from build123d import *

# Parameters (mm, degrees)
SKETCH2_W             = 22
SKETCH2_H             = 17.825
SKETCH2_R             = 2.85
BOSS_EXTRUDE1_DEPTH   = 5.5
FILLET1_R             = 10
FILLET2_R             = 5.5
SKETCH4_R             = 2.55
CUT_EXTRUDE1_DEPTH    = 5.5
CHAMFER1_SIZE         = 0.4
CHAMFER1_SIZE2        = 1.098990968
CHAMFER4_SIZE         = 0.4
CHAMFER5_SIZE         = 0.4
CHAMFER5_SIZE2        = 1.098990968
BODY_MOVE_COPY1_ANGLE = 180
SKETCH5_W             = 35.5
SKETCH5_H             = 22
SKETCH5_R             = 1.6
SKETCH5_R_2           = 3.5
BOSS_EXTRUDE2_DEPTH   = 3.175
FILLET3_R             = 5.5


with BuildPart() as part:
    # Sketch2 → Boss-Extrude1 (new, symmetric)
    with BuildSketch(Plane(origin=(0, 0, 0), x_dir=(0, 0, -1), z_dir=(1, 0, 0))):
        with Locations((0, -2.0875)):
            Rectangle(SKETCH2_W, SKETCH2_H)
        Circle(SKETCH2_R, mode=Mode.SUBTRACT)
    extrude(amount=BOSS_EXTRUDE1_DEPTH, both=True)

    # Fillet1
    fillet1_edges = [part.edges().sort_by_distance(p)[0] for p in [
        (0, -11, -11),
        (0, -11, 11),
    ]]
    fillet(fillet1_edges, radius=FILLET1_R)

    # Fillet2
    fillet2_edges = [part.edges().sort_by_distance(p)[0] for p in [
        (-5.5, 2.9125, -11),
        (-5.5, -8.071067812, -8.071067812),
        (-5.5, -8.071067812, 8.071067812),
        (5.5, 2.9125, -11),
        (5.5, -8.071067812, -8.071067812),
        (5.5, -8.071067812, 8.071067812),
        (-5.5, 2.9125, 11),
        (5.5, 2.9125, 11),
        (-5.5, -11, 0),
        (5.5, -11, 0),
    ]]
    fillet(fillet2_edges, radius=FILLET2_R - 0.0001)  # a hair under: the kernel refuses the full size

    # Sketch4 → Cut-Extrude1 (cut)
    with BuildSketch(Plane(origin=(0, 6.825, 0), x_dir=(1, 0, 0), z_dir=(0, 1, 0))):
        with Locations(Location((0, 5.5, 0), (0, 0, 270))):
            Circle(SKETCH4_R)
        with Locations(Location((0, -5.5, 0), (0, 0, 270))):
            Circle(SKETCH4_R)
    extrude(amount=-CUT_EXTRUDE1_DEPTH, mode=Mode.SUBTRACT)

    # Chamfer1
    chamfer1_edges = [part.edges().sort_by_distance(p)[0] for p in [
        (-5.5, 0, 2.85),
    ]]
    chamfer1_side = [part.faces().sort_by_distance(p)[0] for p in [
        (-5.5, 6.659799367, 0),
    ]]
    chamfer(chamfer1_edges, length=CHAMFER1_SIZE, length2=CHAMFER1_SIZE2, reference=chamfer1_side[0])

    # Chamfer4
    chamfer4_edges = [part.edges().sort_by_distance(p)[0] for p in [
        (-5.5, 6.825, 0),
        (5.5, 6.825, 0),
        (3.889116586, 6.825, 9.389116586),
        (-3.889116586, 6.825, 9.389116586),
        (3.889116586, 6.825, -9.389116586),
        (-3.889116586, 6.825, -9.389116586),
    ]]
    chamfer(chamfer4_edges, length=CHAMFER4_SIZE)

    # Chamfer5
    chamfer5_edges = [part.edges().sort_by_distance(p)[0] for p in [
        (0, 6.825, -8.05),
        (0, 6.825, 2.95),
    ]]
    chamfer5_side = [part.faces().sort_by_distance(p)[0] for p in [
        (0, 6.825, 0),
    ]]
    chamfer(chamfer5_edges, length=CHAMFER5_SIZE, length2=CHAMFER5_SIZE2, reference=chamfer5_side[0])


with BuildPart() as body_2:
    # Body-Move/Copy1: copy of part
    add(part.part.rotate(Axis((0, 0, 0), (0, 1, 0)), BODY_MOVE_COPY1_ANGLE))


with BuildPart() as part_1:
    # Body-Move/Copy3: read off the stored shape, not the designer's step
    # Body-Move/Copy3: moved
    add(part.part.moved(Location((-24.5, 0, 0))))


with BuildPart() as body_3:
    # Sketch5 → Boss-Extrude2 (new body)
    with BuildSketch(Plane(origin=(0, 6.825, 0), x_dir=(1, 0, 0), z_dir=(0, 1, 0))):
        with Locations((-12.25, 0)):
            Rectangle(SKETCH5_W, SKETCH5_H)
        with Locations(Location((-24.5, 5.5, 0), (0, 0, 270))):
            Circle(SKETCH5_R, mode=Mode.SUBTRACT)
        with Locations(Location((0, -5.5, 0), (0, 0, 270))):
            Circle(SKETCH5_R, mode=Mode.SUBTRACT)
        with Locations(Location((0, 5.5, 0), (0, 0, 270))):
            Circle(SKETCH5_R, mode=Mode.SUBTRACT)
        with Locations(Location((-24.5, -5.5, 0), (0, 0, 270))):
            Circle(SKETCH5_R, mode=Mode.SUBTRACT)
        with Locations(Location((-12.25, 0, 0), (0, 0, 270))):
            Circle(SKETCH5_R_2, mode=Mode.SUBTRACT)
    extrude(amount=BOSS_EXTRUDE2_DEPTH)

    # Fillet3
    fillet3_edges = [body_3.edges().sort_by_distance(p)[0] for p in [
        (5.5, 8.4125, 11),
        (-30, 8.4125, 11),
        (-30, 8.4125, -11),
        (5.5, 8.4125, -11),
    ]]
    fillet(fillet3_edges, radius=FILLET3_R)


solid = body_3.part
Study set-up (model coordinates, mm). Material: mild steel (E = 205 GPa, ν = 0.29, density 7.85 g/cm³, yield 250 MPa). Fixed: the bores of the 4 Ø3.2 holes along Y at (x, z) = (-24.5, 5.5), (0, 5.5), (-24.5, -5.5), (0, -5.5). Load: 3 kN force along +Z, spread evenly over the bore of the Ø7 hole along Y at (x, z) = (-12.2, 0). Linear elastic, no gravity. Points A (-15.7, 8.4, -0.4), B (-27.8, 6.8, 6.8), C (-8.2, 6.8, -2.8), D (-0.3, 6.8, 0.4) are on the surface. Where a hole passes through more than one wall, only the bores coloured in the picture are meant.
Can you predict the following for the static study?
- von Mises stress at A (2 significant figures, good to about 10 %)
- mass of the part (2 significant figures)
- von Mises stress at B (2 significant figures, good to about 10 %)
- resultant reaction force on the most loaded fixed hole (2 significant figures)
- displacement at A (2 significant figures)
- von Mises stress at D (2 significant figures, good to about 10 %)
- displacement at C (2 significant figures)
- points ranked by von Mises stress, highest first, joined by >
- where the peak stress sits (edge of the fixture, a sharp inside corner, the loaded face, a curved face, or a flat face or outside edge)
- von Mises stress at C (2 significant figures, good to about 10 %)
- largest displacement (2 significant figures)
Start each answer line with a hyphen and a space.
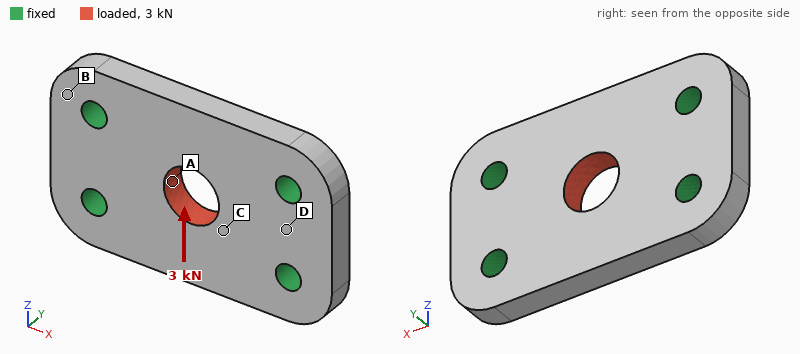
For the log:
- 78 MPa
- 17 g
- 10 MPa
- 880 N
- 3.2 µm
- 19 MPa
- 2.9 µm
- A > C > D > B
- edge of the fixture
- 45 MPa
- 4.0 µm
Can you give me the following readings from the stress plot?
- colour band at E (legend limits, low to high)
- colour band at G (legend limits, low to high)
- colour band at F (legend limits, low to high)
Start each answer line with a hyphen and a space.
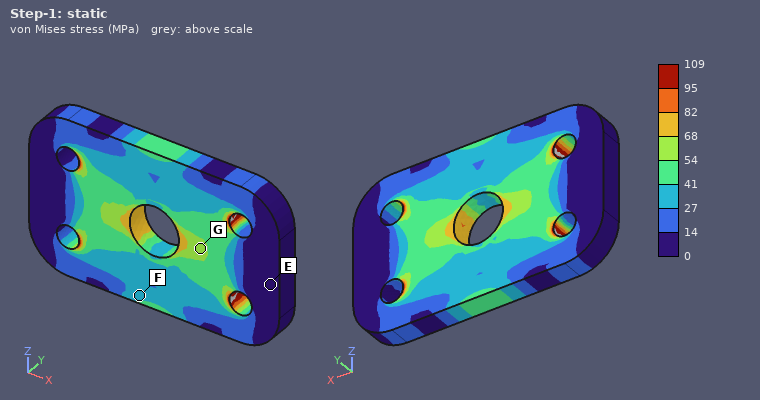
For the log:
- 0 to 14 MPa
- 54 to 68 MPa
- 27 to 41 MPa
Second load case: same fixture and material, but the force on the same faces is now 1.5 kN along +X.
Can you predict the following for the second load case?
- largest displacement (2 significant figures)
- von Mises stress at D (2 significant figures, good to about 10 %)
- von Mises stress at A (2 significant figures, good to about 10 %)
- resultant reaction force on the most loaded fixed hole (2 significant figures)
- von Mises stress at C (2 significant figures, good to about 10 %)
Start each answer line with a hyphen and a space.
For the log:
- 0.92 µm
- 5.9 MPa
- 20 MPa
- 390 N
- 21 MPa
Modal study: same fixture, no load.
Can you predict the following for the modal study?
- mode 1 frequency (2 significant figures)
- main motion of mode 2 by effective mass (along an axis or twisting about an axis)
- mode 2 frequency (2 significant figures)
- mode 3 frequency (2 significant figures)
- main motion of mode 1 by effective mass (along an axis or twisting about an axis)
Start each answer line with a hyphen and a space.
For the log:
- 28 kHz
- twisting about X
- 30 kHz
- 50 kHz
- along Y
